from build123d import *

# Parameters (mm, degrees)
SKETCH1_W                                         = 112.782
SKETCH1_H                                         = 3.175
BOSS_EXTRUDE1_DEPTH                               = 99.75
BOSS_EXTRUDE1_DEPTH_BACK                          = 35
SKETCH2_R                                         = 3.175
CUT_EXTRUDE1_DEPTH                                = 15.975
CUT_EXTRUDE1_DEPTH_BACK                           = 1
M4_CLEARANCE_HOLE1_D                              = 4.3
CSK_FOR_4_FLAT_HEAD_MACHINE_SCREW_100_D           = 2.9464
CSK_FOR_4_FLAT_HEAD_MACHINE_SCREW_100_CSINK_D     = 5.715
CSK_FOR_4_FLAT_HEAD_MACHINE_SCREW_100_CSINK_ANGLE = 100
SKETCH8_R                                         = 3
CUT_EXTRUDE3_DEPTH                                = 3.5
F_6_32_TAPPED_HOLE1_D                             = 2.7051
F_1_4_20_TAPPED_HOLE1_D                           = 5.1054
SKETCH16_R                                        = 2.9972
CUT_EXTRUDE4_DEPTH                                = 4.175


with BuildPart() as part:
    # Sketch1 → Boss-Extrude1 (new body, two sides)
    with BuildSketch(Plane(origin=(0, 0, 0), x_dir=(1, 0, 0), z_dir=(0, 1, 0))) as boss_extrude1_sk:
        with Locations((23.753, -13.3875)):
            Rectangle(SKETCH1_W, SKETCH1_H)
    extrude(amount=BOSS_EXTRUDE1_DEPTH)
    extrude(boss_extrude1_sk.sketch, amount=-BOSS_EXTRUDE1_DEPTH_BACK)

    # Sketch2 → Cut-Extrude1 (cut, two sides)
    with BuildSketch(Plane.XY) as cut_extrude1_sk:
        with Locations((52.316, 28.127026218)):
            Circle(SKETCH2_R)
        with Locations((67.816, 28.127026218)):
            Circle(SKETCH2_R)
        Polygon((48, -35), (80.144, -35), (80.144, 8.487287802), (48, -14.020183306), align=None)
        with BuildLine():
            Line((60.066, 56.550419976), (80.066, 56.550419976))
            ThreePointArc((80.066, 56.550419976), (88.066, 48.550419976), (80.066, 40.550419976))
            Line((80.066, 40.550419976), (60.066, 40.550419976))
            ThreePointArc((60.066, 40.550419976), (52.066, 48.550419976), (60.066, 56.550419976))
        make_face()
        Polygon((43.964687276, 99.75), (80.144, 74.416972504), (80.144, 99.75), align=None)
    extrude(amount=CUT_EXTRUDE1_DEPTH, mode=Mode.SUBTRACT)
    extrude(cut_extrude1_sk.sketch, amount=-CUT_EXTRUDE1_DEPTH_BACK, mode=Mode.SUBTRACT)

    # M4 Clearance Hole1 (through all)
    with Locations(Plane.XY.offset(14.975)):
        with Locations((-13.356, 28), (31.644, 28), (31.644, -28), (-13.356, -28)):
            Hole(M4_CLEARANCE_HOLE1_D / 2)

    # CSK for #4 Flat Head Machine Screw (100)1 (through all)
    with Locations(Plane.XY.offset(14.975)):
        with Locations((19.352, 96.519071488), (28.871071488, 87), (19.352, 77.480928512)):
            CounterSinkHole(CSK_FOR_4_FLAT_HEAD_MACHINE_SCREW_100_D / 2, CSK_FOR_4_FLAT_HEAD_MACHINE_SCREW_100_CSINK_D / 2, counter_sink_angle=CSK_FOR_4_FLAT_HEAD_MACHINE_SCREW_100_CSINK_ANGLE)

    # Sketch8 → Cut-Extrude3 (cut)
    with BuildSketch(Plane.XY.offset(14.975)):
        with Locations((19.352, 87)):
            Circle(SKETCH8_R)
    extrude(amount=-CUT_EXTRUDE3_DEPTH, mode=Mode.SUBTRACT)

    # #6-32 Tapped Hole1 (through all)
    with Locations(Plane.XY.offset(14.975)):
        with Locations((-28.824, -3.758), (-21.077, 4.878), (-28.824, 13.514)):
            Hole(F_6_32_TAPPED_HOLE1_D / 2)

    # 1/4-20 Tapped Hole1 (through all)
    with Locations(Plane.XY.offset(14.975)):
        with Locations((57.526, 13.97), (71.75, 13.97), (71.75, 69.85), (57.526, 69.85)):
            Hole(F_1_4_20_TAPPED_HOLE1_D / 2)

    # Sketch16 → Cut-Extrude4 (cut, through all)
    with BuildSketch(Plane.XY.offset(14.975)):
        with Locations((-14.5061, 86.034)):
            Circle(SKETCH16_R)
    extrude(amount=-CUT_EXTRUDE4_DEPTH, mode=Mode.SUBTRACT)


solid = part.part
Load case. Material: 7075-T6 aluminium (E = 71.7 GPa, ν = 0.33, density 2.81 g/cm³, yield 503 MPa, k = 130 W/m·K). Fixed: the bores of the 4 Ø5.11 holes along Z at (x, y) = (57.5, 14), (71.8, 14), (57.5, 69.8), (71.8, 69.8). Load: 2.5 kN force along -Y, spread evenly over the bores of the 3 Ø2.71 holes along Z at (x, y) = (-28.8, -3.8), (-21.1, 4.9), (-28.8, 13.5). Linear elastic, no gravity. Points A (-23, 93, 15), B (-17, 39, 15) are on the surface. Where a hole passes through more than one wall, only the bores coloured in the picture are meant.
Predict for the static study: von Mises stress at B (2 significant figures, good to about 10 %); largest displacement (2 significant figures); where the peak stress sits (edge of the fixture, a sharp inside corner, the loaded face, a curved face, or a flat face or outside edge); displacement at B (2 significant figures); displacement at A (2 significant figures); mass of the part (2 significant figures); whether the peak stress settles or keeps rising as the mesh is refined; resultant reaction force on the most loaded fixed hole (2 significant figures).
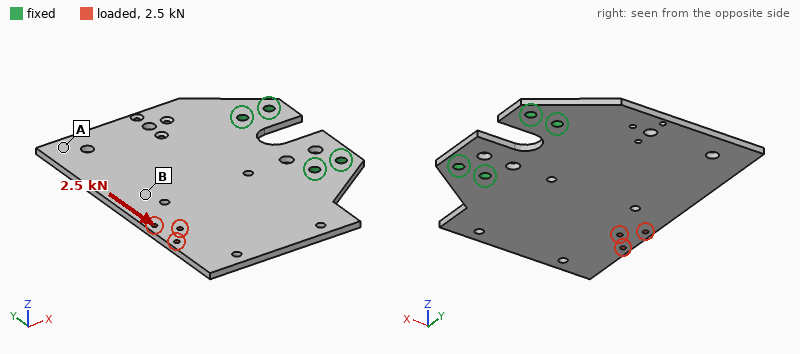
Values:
20 MPa
0.11 mm
edge of the fixture
0.068 mm
0.076 mm
120 g
keeps rising
3.1 kN
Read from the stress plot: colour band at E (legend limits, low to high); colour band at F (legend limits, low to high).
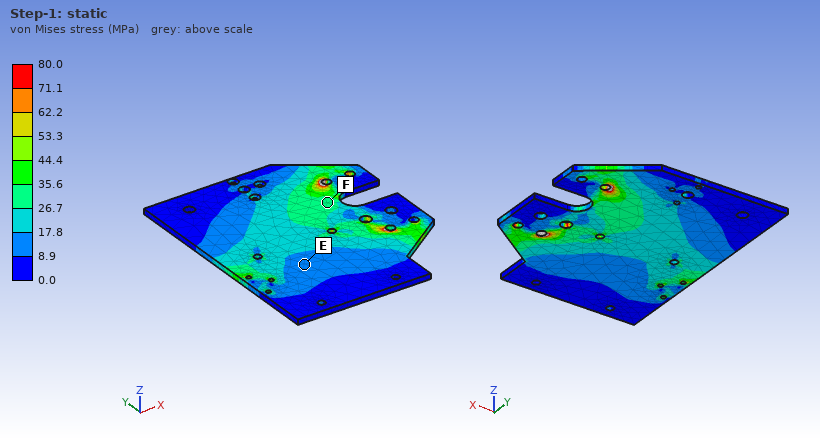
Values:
8.9 to 17.8 MPa
26.7 to 35.6 MPa
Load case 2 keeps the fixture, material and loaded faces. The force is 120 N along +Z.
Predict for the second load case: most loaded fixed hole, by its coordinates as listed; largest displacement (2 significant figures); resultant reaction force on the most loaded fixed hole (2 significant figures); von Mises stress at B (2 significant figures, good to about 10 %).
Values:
(57.5, 14)
1.8 mm
320 N
20 MPa
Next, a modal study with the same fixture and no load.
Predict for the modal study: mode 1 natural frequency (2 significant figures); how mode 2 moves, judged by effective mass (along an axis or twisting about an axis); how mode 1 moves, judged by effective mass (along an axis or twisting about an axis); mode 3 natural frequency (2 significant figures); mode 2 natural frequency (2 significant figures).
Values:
280 Hz
twisting about X
along Z
1100 Hz
480 Hz
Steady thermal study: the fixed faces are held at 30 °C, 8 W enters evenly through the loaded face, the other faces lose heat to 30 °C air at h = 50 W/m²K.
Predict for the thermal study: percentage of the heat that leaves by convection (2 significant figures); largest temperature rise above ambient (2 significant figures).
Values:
66 %
15 K
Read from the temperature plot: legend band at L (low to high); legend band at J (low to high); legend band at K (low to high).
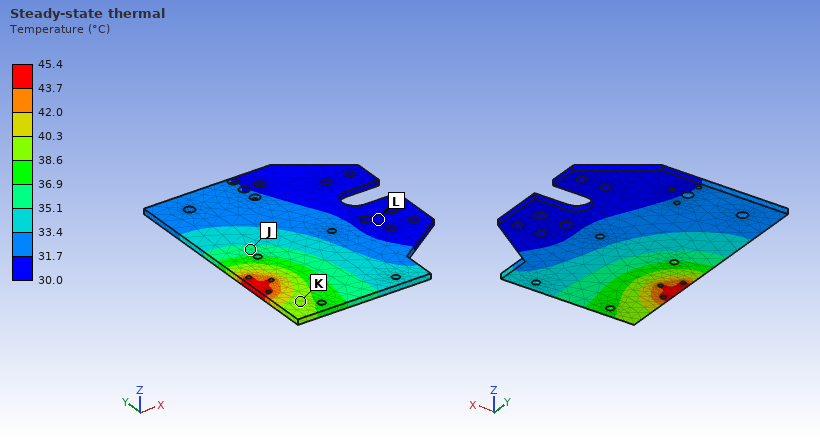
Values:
30.0 to 31.7 °C
35.1 to 36.9 °C
38.6 to 40.3 °C
